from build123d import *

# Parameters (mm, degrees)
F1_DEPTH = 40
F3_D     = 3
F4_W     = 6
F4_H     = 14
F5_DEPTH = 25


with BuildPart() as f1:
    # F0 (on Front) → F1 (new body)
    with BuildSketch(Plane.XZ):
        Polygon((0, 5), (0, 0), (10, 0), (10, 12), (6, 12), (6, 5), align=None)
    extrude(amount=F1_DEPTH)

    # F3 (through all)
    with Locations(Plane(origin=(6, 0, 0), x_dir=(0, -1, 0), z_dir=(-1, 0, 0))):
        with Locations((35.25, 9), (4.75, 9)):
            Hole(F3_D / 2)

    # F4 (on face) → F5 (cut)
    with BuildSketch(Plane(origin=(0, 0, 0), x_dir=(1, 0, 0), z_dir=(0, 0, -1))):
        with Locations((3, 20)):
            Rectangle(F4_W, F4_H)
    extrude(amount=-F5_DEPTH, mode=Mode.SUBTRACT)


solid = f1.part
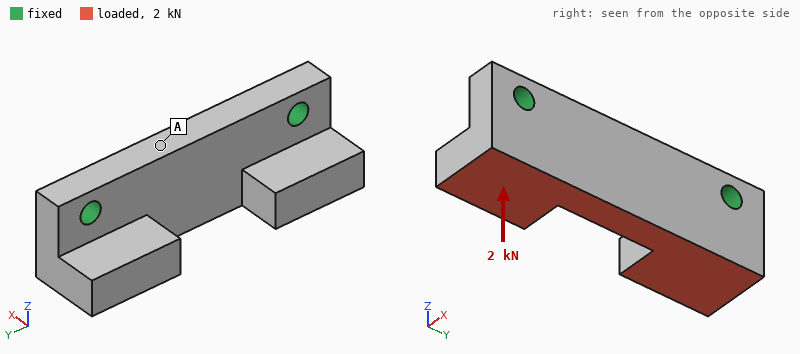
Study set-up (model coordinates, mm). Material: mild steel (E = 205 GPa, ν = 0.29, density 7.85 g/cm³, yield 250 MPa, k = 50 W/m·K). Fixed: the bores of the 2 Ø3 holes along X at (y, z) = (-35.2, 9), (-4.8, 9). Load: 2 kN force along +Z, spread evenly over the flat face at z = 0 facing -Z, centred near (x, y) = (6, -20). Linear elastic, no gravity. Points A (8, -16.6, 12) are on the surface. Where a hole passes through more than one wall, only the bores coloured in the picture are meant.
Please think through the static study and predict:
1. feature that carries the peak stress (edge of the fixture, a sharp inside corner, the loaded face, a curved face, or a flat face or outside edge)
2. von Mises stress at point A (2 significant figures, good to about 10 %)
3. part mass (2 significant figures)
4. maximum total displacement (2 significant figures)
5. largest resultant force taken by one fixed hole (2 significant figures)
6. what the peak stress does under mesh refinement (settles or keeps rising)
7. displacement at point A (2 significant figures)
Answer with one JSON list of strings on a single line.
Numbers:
["edge of the fixture", "16 MPa", "21 g", "13 µm", "1.0 kN", "keeps rising", "3.5 µm"]
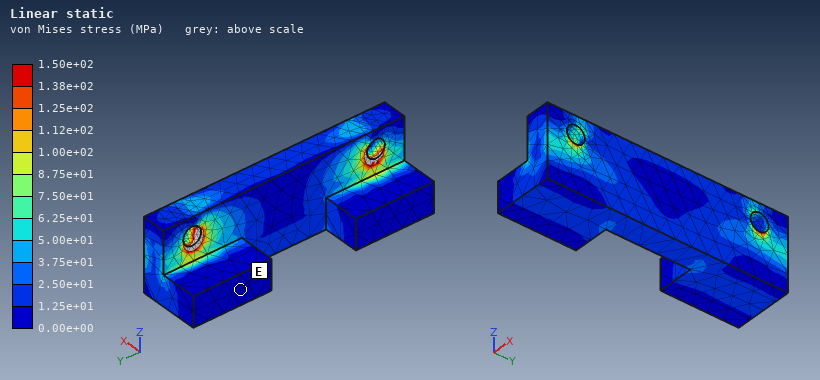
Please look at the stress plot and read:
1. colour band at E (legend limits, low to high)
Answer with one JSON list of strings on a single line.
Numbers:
["0.00e+00 to 1.25e+01 MPa"]
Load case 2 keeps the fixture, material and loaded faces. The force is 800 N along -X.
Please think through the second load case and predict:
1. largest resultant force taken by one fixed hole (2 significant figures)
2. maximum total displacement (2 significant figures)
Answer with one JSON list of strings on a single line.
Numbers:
["400 N", "14 µm"]
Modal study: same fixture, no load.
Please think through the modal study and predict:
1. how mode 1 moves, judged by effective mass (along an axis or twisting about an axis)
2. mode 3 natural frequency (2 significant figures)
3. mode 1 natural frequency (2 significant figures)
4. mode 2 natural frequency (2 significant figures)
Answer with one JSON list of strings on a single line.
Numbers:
["along X", "21 kHz", "14 kHz", "20 kHz"]
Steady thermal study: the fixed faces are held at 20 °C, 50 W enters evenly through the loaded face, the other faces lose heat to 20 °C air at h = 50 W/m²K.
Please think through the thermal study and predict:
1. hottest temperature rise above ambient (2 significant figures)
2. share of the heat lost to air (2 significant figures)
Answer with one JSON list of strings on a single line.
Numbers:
["76 K", "6.6 %"]
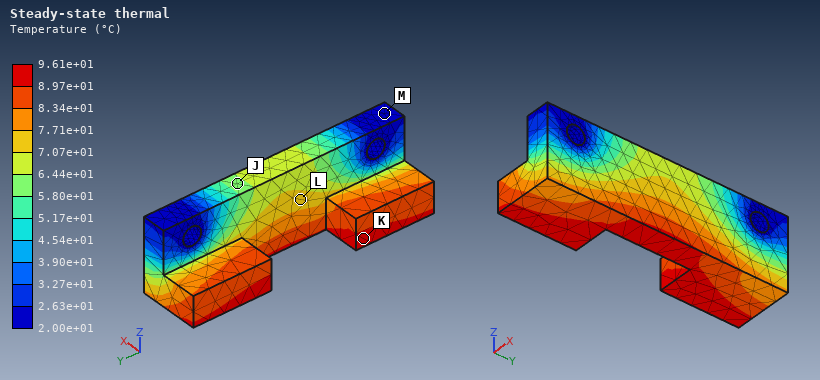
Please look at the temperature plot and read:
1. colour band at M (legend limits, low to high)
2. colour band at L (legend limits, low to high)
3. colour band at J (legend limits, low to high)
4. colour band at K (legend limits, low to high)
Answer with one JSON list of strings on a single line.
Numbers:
["2.00e+01 to 2.63e+01 °C", "7.07e+01 to 7.71e+01 °C", "5.80e+01 to 6.44e+01 °C", "8.97e+01 to 9.61e+01 °C"]
